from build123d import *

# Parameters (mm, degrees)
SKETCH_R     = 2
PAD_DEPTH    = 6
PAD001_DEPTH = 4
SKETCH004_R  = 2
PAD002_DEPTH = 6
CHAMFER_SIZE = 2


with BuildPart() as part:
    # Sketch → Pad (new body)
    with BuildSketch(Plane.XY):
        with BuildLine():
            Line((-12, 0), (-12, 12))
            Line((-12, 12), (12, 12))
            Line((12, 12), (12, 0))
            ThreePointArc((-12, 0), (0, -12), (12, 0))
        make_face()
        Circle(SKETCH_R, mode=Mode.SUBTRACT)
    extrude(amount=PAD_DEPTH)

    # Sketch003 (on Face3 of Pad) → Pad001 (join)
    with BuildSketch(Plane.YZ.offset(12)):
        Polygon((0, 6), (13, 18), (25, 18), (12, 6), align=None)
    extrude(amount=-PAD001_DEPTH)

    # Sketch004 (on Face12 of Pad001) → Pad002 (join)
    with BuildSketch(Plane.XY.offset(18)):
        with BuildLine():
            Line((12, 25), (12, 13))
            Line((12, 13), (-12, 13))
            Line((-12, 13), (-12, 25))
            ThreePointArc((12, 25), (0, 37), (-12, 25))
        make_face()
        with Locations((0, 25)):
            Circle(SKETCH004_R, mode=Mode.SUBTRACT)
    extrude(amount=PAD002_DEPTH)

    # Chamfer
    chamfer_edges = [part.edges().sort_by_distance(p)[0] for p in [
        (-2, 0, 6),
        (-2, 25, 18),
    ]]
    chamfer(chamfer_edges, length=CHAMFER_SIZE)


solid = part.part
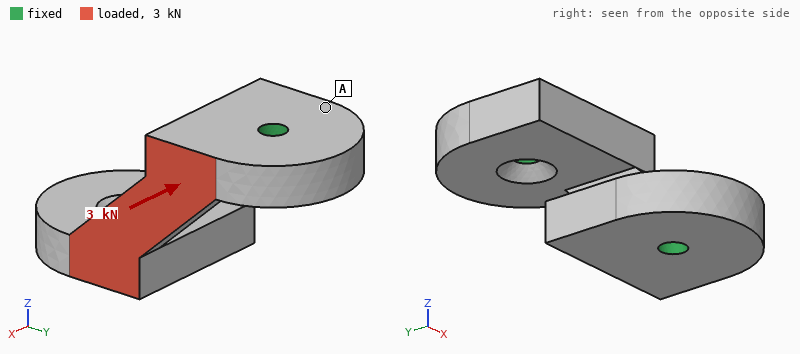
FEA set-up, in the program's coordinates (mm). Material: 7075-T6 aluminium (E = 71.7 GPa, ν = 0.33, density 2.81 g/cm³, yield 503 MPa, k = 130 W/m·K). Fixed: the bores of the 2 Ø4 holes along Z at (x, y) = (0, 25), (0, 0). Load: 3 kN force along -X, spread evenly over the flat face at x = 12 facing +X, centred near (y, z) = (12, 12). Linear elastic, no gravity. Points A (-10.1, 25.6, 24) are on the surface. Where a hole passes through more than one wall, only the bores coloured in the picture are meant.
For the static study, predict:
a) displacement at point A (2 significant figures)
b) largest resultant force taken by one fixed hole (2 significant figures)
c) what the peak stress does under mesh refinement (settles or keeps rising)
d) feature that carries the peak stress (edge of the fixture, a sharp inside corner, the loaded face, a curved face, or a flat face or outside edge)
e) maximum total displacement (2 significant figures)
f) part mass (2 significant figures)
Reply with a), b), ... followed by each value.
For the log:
a) 7.2 µm
b) 1.7 kN
c) keeps rising
d) edge of the fixture
e) 23 µm
f) 18 g
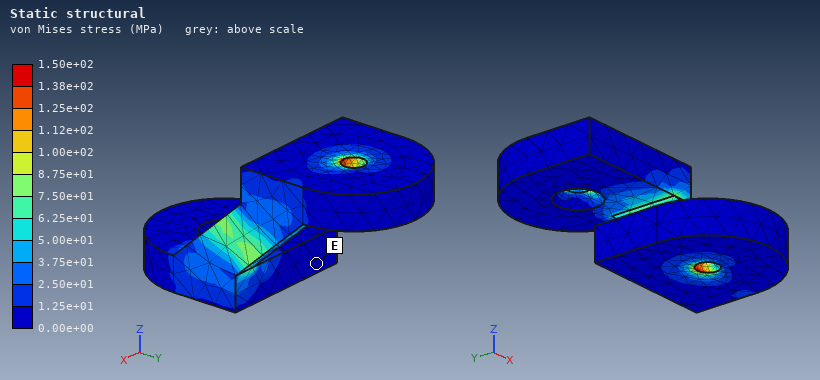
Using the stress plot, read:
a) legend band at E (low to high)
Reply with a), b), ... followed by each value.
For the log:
a) 0.00e+00 to 1.25e+01 MPa
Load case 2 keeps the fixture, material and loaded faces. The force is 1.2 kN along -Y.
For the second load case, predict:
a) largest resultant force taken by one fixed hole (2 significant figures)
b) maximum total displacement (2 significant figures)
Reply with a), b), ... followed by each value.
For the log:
a) 610 N
b) 24 µm
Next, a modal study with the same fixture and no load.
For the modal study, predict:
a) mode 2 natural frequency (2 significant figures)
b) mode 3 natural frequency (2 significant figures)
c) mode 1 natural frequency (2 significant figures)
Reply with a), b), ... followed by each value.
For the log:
a) 17 kHz
b) 17 kHz
c) 14 kHz
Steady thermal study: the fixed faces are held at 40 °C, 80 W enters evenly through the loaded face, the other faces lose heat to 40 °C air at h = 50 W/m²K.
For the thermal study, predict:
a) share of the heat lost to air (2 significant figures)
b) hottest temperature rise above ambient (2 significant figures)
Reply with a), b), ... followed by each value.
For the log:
a) 3.2 %
b) 62 K
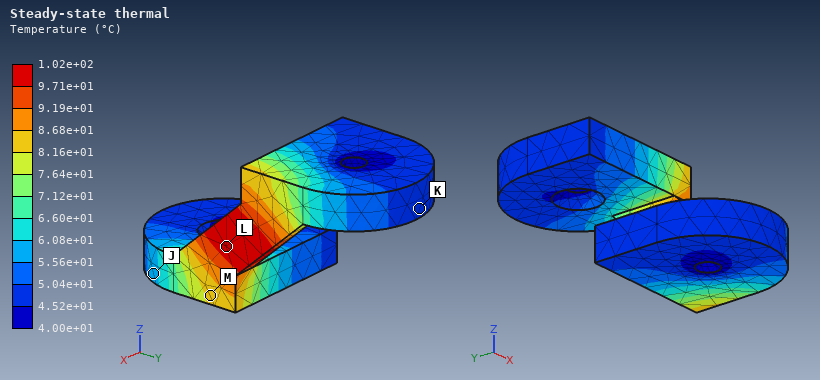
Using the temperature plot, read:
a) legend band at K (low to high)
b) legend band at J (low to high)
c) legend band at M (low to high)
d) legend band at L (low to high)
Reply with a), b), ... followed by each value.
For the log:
a) 4.52e+01 to 5.04e+01 °C
b) 5.56e+01 to 6.08e+01 °C
c) 8.16e+01 to 8.68e+01 °C
d) 9.71e+01 to 1.02e+02 °C
